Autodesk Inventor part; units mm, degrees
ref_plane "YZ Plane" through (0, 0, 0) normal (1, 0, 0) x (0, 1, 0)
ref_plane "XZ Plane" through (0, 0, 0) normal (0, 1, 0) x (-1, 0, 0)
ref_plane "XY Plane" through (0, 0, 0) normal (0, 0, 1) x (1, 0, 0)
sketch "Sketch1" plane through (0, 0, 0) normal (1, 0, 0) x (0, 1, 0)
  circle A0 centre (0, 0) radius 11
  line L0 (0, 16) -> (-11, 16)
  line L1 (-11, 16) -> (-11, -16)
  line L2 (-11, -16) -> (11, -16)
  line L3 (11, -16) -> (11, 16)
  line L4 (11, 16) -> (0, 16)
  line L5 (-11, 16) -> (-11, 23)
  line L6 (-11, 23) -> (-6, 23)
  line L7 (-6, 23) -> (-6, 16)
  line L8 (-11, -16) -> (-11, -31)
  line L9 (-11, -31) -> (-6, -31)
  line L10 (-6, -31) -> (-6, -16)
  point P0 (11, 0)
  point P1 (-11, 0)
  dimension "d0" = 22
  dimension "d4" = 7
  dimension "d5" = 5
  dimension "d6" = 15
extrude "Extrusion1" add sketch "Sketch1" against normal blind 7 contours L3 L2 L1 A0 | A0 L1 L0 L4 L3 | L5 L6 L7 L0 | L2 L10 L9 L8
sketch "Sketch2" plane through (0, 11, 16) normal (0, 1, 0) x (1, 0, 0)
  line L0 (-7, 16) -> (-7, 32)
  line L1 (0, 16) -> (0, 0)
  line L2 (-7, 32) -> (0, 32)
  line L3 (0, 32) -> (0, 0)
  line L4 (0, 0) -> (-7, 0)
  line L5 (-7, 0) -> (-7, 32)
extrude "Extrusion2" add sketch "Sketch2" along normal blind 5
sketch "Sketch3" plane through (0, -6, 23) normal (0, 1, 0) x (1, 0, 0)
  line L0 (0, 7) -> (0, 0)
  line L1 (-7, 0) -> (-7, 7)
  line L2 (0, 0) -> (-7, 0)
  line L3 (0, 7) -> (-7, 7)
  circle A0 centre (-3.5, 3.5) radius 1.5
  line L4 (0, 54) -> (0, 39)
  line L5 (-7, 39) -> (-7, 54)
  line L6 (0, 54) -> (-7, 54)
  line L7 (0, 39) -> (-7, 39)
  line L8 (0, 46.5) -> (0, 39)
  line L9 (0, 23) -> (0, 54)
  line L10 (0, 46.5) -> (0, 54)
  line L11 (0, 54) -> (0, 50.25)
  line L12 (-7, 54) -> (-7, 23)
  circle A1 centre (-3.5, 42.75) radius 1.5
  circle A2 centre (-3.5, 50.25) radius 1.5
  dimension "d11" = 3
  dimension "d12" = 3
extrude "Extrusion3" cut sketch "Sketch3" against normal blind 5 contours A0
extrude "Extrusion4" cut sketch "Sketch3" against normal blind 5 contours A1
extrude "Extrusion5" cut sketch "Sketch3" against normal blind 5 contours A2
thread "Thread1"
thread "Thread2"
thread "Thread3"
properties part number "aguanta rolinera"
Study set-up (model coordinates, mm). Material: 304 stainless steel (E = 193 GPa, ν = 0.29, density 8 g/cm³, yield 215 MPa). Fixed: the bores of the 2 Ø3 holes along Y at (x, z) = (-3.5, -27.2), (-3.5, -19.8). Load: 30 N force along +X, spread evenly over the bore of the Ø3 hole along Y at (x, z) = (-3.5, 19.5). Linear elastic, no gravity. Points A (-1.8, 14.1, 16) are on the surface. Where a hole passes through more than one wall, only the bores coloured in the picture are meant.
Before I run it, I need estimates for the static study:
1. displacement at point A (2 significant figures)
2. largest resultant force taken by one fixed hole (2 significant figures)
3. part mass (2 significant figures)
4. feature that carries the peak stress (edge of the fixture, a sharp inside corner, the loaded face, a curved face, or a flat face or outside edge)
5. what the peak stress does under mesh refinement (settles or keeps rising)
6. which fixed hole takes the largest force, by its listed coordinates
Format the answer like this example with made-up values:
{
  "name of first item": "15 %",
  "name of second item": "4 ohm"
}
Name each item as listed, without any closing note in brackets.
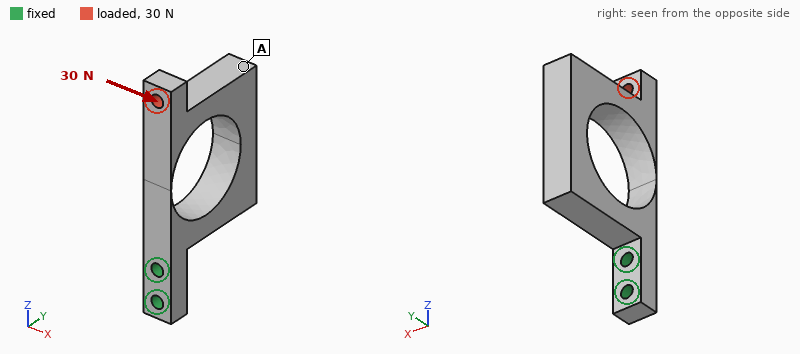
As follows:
{
  "displacement at point A": "34 µm",
  "largest resultant force taken by one fixed hole": "75 N",
  "part mass": "32 g",
  "feature that carries the peak stress": "a sharp inside corner",
  "what the peak stress does under mesh refinement": "keeps rising",
  "which fixed hole takes the largest force, by its listed coordinates": "(-3.5, -19.8)"
}
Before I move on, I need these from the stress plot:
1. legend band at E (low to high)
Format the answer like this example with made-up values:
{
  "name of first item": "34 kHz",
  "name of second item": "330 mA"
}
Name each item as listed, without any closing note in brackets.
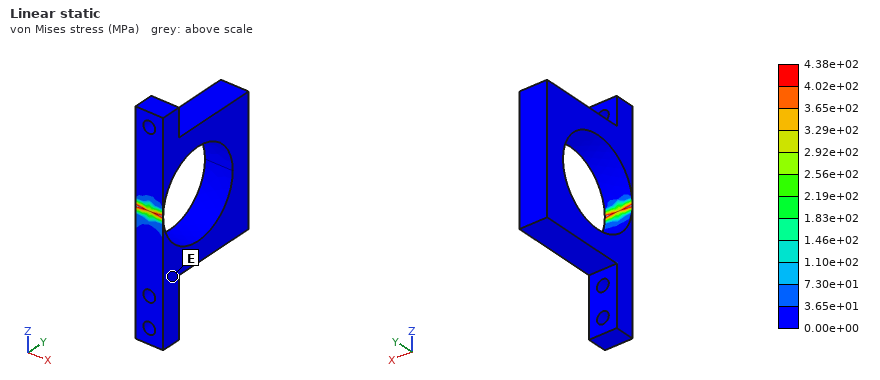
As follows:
{
  "legend band at E": "0.00e+00 to 3.65e+01 MPa"
}
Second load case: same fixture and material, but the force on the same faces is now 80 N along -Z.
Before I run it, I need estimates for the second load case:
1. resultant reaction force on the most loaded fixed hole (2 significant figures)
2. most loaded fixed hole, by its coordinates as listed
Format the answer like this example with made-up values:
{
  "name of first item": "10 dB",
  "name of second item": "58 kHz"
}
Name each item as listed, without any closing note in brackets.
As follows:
{
  "resultant reaction force on the most loaded fixed hole": "75 N",
  "most loaded fixed hole, by its coordinates as listed": "(-3.5, -19.8)"
}
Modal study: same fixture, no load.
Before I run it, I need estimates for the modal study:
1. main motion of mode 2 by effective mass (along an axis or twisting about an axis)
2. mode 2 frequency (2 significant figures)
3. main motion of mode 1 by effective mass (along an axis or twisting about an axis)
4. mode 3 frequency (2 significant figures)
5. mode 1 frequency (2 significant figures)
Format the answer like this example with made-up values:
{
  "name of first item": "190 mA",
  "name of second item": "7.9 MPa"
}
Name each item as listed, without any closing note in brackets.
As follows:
{
  "main motion of mode 2 by effective mass": "along X",
  "mode 2 frequency": "1400 Hz",
  "main motion of mode 1 by effective mass": "along Y",
  "mode 3 frequency": "3000 Hz",
  "mode 1 frequency": "1300 Hz"
}
